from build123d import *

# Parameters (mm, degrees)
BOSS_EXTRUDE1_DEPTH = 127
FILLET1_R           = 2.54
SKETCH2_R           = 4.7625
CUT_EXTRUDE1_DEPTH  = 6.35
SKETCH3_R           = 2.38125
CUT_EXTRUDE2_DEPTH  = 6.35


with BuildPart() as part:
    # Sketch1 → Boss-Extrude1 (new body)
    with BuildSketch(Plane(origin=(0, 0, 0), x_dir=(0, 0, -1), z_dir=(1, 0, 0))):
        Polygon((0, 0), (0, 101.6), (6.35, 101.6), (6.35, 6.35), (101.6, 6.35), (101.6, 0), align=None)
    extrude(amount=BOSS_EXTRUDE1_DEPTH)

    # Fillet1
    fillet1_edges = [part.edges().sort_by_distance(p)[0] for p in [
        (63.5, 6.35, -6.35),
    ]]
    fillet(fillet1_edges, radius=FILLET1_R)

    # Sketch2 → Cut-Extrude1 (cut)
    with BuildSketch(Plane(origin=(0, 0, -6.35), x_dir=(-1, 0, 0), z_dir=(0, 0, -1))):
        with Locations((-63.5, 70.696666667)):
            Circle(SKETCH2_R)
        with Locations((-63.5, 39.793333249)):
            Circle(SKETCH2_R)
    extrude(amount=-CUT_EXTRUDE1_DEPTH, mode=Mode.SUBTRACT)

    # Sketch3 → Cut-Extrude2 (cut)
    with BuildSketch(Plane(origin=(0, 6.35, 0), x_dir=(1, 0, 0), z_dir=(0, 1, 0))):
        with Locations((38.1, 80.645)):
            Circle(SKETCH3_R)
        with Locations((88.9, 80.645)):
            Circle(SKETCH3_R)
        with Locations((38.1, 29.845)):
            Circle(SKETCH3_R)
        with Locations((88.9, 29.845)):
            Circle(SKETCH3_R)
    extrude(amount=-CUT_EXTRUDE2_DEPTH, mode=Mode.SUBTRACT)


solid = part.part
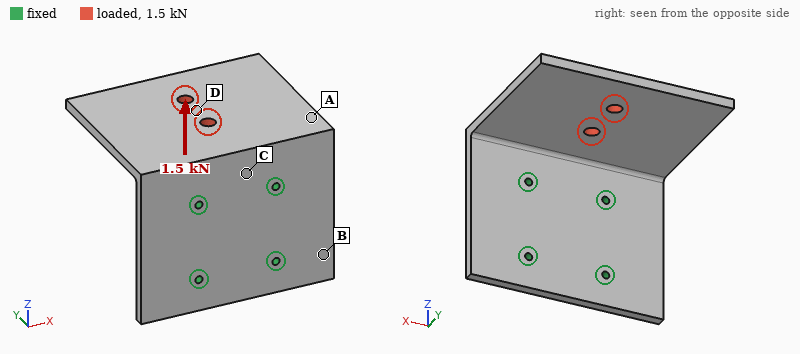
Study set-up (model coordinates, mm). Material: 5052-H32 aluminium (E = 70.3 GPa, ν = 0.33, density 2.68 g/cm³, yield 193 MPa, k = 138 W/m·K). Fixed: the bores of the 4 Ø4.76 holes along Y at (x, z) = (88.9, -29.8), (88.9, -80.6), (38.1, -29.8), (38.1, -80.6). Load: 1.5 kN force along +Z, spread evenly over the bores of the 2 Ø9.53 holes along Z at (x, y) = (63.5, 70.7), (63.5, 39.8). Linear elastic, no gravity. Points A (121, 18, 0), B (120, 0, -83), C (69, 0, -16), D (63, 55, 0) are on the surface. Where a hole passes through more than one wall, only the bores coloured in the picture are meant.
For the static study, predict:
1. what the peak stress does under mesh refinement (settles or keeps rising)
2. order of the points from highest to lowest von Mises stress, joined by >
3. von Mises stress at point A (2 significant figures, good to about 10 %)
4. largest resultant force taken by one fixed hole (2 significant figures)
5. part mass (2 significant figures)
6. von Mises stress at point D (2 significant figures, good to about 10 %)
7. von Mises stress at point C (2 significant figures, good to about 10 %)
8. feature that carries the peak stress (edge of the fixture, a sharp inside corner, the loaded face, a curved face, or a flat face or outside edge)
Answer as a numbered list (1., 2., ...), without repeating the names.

1. keeps rising
2. C > A > D > B
3. 60 MPa
4. 740 N
5. 420 g
6. 32 MPa
7. 85 MPa
8. edge of the fixture
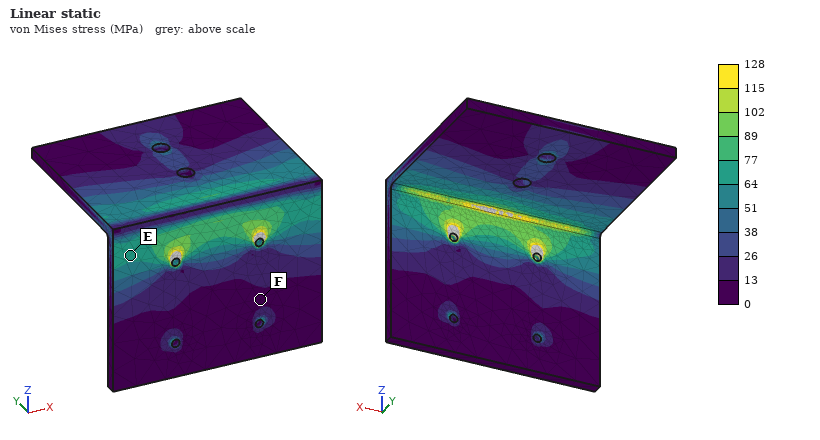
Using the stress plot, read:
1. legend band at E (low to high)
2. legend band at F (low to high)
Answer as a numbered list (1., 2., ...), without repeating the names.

1. 64 to 77 MPa
2. 0 to 13 MPa
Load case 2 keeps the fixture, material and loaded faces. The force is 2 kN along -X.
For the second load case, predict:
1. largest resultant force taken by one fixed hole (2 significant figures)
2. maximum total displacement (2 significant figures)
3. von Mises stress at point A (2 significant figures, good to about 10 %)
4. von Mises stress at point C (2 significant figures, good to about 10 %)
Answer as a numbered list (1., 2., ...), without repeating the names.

1. 2.2 kN
2. 0.41 mm
3. 20 MPa
4. 30 MPa
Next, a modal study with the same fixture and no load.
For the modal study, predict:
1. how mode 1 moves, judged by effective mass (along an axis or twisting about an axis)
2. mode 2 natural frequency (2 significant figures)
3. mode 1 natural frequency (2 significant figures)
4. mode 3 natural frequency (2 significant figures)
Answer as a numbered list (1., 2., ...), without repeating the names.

1. along Z
2. 800 Hz
3. 380 Hz
4. 1200 Hz
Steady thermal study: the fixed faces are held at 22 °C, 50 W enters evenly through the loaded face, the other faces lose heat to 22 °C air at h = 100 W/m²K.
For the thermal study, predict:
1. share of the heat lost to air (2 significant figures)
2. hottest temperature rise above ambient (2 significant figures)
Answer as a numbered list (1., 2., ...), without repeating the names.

1. 70 %
2. 23 K
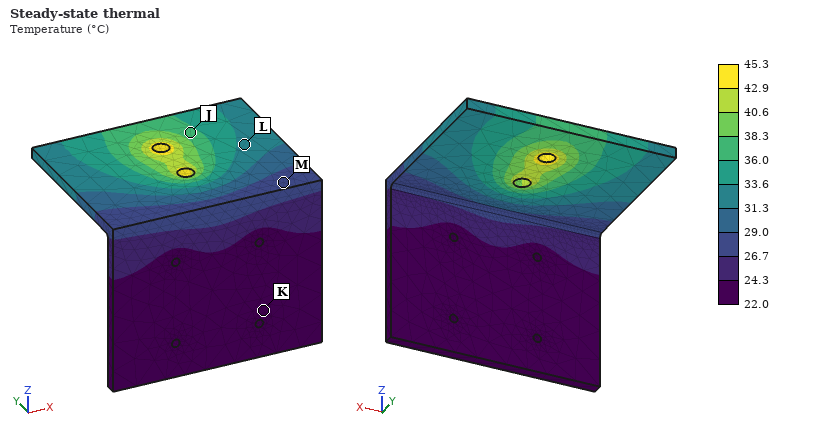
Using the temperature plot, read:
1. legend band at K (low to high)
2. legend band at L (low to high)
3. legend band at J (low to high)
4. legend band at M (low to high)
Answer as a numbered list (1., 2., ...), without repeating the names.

1. 22.0 to 24.3 °C
2. 31.3 to 33.6 °C
3. 36.0 to 38.3 °C
4. 26.7 to 29.0 °C
